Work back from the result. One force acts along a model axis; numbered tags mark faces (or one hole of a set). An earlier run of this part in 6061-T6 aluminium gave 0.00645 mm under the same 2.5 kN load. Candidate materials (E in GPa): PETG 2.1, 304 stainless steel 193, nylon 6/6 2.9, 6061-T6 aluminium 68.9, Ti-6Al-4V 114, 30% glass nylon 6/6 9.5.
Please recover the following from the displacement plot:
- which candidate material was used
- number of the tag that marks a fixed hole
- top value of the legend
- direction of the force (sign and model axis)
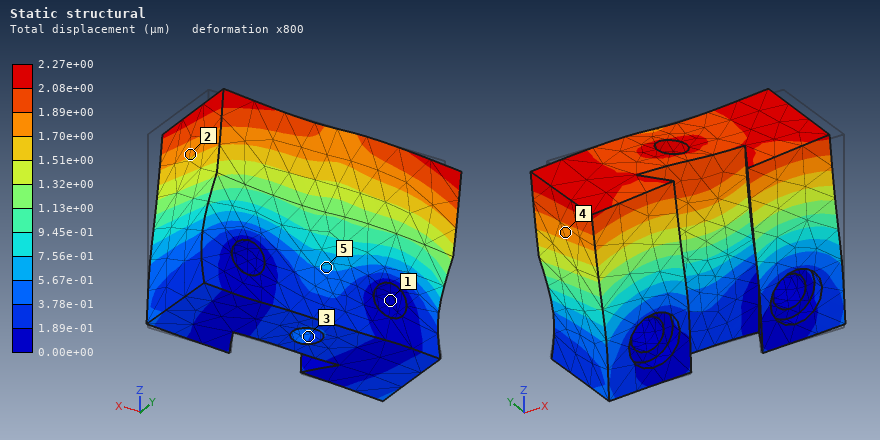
304 stainless steel
1
2.27e+00 µm
-X
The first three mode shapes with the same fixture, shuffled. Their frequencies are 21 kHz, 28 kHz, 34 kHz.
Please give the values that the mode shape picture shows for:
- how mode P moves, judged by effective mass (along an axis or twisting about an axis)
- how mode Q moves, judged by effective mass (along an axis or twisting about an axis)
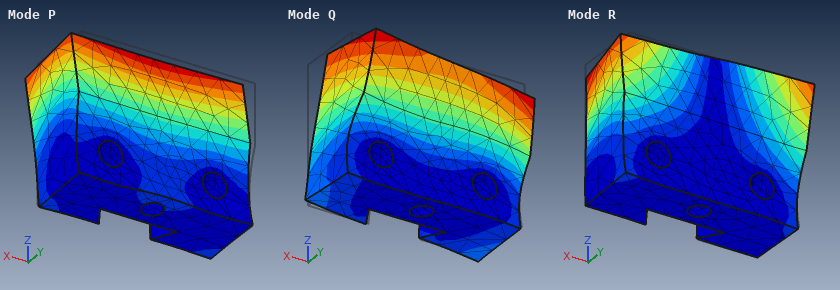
along Y
along X
